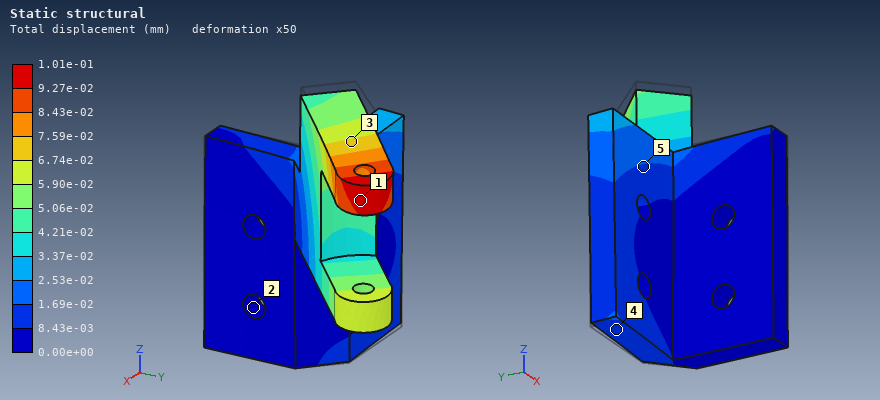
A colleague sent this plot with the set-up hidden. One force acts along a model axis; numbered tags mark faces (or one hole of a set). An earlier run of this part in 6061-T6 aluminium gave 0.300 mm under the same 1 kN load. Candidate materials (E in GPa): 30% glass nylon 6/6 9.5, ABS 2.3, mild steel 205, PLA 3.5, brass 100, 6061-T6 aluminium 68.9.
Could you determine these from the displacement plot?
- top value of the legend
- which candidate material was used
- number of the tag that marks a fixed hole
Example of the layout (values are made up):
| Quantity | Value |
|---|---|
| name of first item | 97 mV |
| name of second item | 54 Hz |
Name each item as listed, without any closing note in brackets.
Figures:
| Quantity | Value |
|---|---|
| top value of the legend | 1.01e-01 mm |
| which candidate material was used | mild steel |
| number of the tag that marks a fixed hole | 2 |
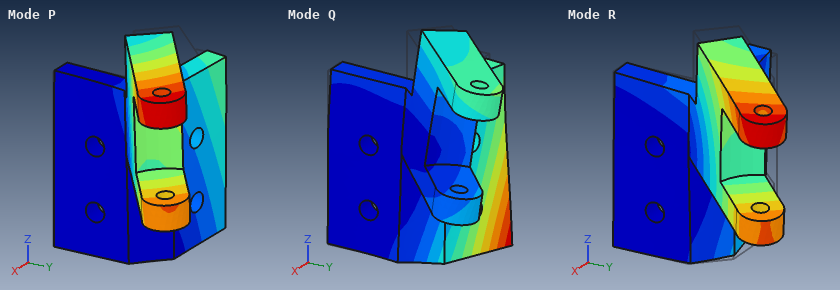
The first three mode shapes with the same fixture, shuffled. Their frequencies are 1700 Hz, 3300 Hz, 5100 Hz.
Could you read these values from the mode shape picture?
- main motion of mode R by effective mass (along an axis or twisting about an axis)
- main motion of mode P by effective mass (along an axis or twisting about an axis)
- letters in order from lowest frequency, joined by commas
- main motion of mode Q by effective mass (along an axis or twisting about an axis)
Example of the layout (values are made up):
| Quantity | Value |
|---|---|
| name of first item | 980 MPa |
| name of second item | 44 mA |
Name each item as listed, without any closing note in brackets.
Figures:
| Quantity | Value |
|---|---|
| main motion of mode R by effective mass | along Z |
| main motion of mode P by effective mass | along X |
| letters in order from lowest frequency, joined by commas | P, R, Q |
| main motion of mode Q by effective mass | along Y |
